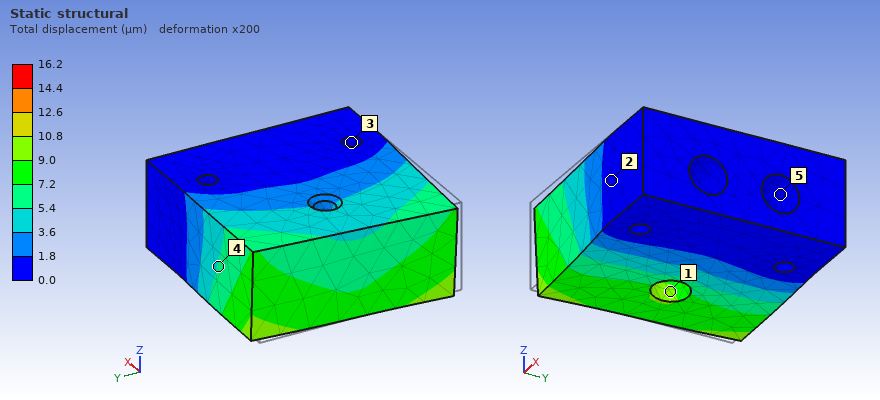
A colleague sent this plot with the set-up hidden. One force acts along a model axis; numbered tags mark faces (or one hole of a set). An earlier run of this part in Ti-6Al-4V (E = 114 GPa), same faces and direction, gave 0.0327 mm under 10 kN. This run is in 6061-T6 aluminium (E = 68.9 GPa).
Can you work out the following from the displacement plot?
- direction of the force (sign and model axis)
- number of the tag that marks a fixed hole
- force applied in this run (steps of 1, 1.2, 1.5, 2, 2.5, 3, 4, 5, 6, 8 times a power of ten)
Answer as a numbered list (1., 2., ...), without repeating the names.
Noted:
1. +Y
2. 3
3. 3 kN
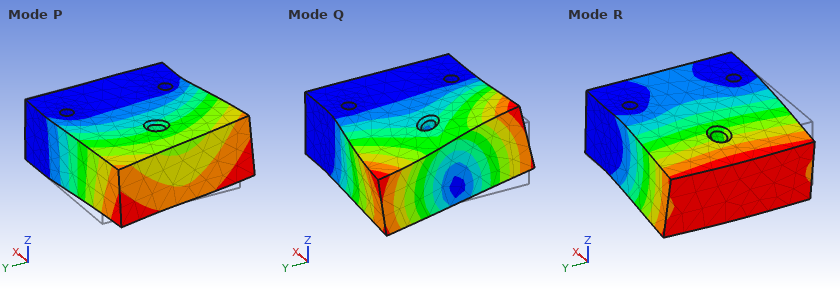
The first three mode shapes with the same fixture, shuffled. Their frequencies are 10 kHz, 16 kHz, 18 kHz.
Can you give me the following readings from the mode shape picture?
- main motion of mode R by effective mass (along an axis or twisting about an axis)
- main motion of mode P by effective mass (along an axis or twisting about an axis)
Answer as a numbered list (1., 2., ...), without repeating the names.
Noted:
1. along Z
2. along Y
